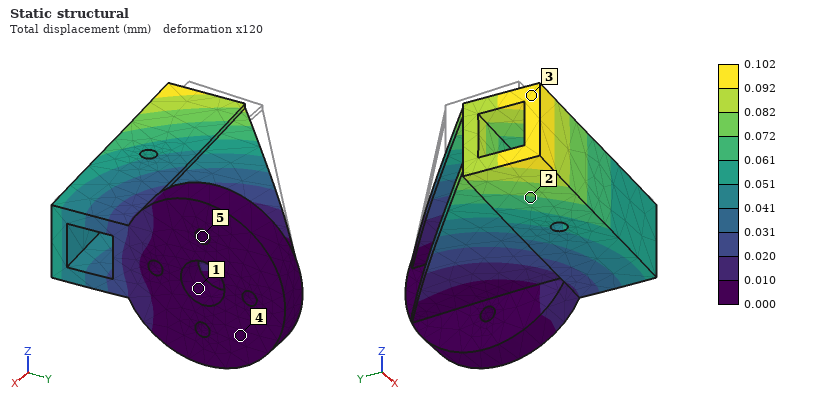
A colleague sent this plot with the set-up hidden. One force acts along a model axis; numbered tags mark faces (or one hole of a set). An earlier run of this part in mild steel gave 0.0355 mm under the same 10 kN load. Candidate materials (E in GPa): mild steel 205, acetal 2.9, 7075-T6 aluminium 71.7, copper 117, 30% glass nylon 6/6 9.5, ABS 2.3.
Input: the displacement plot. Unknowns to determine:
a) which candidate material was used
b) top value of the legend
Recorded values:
7075-T6 aluminium
0.102 mm
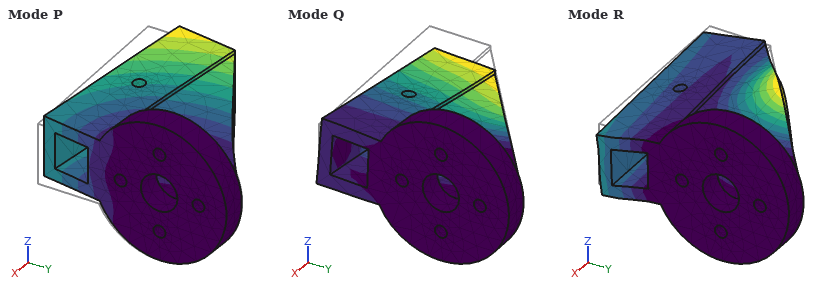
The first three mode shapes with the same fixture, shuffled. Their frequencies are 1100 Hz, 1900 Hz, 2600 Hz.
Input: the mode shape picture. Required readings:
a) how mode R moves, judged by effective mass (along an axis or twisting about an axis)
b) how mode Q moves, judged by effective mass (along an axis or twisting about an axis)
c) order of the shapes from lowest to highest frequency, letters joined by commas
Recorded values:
twisting about X
along Z
Q, P, R
